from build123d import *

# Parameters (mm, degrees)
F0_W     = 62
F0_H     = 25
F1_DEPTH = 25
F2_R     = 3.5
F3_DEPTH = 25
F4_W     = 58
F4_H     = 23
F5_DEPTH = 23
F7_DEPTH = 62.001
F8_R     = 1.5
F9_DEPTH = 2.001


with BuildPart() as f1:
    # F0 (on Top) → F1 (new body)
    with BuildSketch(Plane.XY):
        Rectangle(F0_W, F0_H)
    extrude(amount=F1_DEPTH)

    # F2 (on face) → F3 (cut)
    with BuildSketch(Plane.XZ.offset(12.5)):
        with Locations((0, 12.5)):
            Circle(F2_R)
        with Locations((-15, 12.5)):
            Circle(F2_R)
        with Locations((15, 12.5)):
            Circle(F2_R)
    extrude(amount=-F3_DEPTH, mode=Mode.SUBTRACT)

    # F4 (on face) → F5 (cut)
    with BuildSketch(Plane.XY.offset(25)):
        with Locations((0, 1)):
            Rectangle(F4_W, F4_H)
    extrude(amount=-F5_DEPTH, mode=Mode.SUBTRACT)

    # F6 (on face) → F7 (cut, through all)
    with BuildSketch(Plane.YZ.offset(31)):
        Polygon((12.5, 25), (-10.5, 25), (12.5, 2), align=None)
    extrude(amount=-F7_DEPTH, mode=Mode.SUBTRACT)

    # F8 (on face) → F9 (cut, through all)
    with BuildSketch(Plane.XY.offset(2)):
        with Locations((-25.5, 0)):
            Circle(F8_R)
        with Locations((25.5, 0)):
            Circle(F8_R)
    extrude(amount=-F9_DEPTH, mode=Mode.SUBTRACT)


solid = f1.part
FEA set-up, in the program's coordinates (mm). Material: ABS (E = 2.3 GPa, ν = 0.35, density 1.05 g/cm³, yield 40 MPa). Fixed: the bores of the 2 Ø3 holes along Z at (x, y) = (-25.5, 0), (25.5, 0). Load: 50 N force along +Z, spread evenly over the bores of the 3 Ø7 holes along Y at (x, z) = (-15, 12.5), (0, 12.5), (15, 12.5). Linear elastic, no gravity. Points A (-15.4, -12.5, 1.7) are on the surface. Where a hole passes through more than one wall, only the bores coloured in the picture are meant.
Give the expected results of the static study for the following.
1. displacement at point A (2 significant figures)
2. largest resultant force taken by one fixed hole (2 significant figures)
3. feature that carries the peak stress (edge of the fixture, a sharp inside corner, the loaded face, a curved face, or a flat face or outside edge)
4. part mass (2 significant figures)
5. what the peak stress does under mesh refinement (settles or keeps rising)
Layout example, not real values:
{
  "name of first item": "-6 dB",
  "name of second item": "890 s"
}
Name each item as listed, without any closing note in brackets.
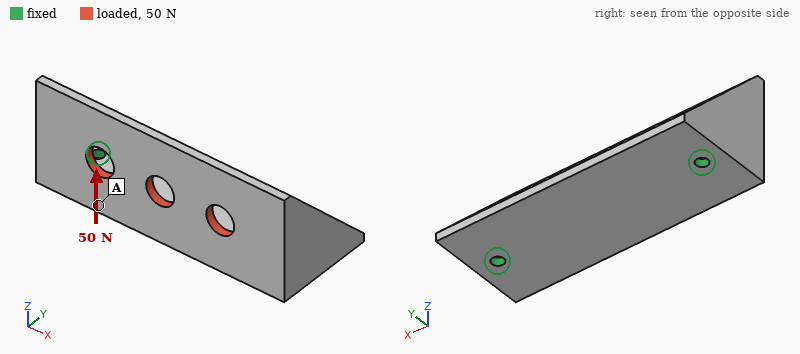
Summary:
{
  "displacement at point A": "0.26 mm",
  "largest resultant force taken by one fixed hole": "25 N",
  "feature that carries the peak stress": "edge of the fixture",
  "part mass": "7.1 g",
  "what the peak stress does under mesh refinement": "keeps rising"
}
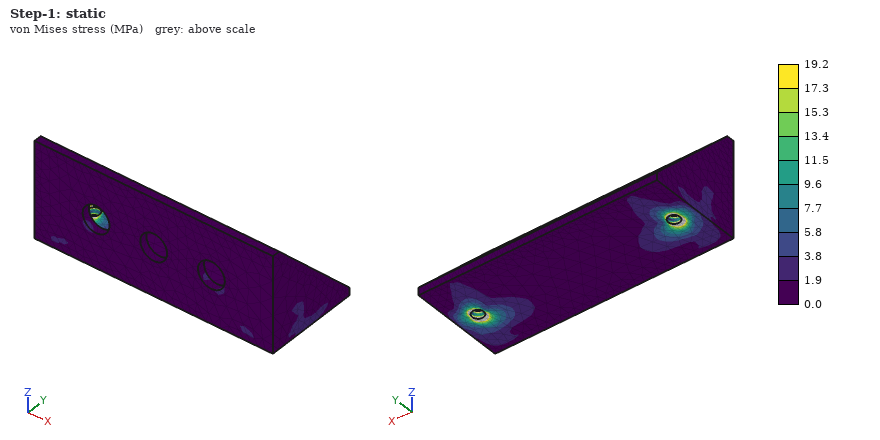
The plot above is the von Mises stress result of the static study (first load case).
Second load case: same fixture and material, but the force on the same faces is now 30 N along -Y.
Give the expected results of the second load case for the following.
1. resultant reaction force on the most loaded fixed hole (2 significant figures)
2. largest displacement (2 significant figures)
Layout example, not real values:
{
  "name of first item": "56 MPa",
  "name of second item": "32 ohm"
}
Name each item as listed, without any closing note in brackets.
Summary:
{
  "resultant reaction force on the most loaded fixed hole": "16 N",
  "largest displacement": "0.78 mm"
}
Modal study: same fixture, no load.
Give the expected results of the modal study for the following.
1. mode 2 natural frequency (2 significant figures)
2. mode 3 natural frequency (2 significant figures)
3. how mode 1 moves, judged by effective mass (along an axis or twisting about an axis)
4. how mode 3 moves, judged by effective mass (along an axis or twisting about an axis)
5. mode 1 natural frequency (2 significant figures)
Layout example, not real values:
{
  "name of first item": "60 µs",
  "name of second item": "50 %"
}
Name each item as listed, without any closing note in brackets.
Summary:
{
  "mode 2 natural frequency": "1100 Hz",
  "mode 3 natural frequency": "1300 Hz",
  "how mode 1 moves, judged by effective mass": "along Y",
  "how mode 3 moves, judged by effective mass": "along Z",
  "mode 1 natural frequency": "700 Hz"
}
